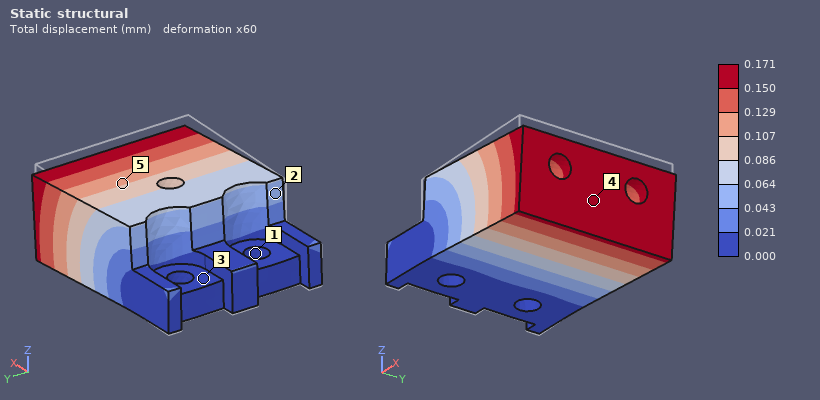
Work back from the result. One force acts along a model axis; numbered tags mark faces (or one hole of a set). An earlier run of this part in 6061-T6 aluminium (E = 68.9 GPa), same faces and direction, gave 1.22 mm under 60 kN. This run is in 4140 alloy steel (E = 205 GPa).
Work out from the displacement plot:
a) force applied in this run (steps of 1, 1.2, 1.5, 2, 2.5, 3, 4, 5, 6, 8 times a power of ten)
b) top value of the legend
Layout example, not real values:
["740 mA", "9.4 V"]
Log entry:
["25 kN", "0.171 mm"]
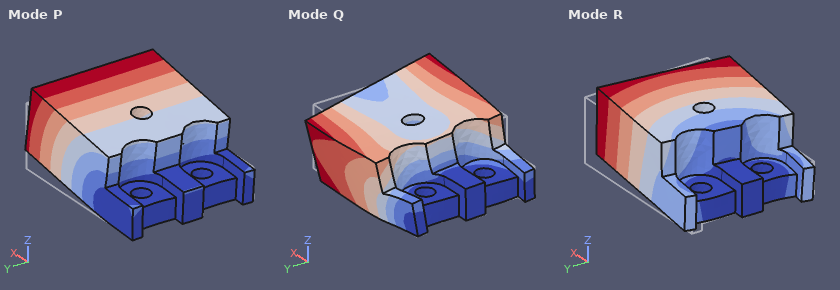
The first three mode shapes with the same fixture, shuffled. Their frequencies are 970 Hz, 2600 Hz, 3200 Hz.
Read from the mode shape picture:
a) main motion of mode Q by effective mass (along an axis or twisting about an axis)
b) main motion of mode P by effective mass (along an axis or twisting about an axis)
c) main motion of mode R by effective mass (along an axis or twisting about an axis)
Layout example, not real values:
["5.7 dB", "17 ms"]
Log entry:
["twisting about X", "along Z", "along Y"]
